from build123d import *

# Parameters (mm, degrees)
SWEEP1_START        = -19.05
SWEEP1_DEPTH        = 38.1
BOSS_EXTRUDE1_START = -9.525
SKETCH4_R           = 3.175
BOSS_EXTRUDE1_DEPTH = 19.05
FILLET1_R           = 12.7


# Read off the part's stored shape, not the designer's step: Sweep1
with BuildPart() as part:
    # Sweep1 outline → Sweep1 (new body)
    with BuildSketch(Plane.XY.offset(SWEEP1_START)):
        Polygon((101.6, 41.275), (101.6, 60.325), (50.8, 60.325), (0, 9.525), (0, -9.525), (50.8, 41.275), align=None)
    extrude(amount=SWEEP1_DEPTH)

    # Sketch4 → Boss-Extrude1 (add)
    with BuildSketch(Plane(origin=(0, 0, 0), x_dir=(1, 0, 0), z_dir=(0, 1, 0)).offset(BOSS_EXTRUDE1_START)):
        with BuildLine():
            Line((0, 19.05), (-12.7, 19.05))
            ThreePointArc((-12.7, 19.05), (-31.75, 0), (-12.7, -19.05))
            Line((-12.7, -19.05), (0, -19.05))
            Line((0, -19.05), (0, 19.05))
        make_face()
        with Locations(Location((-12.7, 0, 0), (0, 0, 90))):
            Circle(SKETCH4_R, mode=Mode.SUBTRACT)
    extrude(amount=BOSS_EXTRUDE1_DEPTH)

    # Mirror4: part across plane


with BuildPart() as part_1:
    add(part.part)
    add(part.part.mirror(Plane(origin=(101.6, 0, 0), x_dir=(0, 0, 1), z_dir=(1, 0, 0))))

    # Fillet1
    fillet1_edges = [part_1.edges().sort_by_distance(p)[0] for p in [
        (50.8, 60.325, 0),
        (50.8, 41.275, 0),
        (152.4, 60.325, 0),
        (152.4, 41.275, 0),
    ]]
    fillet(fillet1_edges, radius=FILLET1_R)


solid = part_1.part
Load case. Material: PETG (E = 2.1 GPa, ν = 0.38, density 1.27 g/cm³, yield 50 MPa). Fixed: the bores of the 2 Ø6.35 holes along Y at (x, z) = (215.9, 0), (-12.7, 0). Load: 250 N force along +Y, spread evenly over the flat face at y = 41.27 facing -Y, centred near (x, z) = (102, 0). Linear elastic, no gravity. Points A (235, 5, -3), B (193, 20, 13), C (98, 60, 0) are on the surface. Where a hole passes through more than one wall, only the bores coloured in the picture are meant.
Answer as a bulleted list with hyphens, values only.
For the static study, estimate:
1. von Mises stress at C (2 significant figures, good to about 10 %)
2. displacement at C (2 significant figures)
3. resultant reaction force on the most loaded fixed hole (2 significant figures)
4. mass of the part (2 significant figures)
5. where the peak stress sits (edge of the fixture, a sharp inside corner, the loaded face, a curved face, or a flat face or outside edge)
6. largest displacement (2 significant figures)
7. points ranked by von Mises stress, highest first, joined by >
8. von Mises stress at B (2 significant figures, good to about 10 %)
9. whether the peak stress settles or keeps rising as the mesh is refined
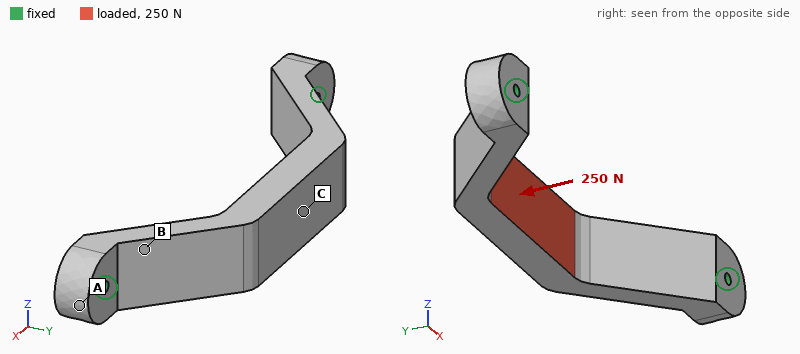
- 1.2 MPa
- 83 µm
- 200 N
- 240 g
- edge of the fixture
- 88 µm
- C > B > A
- 0.45 MPa
- keeps rising
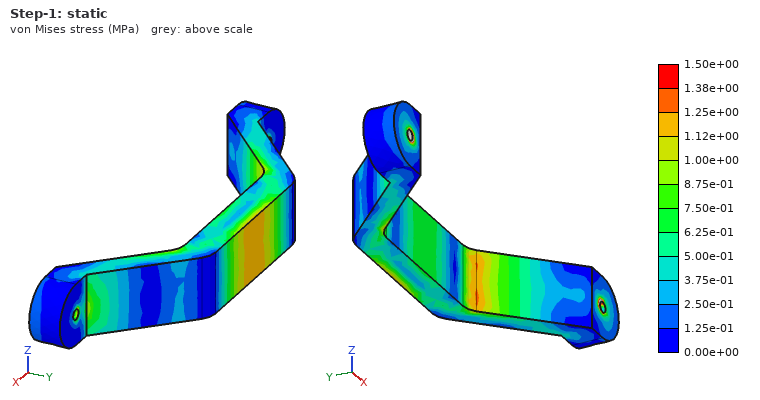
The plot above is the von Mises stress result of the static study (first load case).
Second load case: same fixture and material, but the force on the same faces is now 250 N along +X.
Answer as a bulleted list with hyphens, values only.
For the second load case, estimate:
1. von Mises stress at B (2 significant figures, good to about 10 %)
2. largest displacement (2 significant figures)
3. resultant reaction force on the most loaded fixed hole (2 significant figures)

- 0.78 MPa
- 0.12 mm
- 130 N
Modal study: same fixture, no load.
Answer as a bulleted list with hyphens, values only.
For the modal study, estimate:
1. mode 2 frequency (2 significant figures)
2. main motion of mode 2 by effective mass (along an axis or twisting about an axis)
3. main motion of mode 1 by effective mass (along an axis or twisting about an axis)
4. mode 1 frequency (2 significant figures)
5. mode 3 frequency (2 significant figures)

- 630 Hz
- along X
- along Z
- 320 Hz
- 930 Hz
